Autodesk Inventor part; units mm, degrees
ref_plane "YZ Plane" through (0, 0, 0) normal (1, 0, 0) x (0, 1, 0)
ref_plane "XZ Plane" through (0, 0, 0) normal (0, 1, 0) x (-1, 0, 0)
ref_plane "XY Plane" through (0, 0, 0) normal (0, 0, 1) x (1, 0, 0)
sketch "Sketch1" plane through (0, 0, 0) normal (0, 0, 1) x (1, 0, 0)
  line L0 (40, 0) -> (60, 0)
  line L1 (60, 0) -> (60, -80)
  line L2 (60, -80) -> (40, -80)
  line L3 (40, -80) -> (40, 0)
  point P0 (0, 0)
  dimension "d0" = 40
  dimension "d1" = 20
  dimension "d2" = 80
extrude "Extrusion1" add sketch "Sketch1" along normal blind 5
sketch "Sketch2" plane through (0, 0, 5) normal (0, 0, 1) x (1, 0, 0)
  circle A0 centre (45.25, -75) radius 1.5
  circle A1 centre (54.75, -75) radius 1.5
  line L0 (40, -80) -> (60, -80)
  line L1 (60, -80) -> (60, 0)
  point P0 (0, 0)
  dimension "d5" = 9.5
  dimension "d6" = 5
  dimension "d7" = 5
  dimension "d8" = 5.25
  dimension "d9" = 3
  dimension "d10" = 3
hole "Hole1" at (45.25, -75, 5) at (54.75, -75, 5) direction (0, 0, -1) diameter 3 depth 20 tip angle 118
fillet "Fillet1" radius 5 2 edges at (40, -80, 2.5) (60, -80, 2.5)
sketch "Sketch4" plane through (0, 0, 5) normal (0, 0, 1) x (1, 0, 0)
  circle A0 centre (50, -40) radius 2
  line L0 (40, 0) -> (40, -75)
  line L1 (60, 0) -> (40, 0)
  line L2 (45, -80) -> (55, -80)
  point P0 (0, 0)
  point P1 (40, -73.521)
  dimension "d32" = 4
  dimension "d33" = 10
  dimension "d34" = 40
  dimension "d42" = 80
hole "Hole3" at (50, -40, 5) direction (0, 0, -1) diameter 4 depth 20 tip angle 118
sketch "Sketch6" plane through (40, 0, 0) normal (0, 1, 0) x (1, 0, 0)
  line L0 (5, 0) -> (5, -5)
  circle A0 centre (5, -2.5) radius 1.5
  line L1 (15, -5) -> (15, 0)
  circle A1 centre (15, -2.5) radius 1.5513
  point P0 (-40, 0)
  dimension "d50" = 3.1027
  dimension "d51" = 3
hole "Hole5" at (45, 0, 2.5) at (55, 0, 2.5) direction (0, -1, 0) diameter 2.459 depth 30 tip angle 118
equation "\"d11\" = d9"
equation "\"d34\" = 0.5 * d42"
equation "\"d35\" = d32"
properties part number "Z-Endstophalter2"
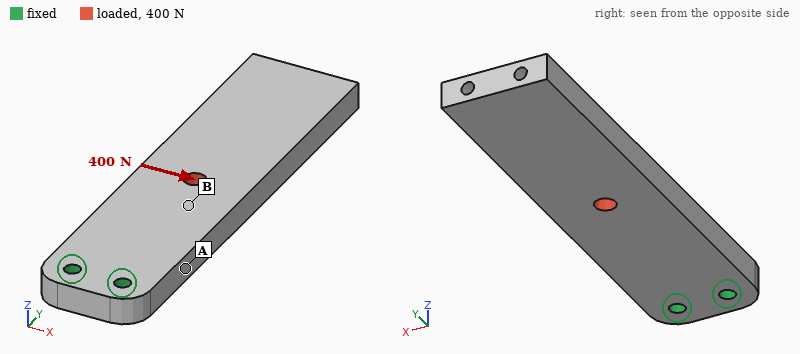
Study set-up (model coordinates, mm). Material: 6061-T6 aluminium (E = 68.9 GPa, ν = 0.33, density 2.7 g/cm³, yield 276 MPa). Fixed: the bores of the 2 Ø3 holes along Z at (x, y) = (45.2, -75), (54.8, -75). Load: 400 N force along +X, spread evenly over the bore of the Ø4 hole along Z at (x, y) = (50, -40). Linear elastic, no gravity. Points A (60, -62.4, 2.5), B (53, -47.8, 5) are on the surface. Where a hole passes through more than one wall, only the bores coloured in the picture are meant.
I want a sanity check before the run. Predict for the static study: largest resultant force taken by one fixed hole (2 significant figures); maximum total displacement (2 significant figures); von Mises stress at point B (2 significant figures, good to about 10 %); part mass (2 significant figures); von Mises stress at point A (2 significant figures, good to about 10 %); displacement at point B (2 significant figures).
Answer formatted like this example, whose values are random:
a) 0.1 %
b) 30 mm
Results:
a) 1.2 kN
b) 86 µm
c) 9.9 MPa
d) 20 g
e) 27 MPa
f) 26 µm
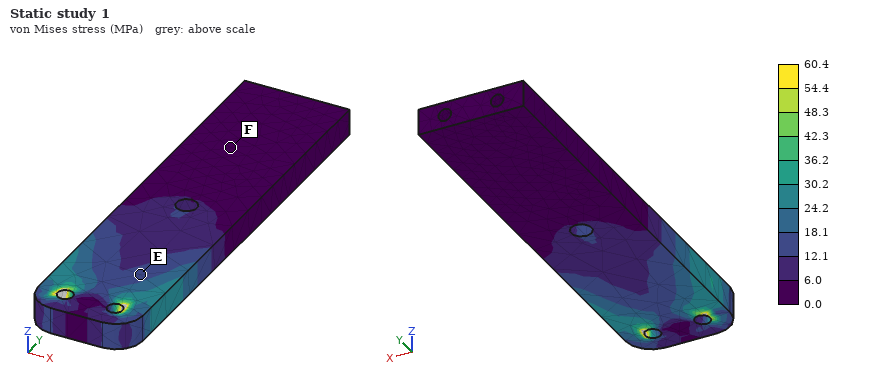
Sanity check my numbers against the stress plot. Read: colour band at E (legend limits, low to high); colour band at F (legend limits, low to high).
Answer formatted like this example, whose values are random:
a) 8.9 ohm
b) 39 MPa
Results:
a) 12.1 to 18.1 MPa
b) 0.0 to 6.0 MPa
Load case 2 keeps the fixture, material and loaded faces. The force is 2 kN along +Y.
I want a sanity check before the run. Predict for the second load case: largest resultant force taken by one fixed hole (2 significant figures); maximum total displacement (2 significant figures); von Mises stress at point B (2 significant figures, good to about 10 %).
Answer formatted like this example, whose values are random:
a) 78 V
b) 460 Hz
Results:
a) 1.0 kN
b) 13 µm
c) 24 MPa
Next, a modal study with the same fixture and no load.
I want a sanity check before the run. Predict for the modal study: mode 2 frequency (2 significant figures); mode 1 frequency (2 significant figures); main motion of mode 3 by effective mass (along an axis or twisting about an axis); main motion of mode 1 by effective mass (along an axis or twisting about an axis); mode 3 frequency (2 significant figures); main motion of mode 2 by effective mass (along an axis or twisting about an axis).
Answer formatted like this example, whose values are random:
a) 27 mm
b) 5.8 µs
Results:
a) 2700 Hz
b) 760 Hz
c) along Z
d) along Z
e) 4500 Hz
f) along X
